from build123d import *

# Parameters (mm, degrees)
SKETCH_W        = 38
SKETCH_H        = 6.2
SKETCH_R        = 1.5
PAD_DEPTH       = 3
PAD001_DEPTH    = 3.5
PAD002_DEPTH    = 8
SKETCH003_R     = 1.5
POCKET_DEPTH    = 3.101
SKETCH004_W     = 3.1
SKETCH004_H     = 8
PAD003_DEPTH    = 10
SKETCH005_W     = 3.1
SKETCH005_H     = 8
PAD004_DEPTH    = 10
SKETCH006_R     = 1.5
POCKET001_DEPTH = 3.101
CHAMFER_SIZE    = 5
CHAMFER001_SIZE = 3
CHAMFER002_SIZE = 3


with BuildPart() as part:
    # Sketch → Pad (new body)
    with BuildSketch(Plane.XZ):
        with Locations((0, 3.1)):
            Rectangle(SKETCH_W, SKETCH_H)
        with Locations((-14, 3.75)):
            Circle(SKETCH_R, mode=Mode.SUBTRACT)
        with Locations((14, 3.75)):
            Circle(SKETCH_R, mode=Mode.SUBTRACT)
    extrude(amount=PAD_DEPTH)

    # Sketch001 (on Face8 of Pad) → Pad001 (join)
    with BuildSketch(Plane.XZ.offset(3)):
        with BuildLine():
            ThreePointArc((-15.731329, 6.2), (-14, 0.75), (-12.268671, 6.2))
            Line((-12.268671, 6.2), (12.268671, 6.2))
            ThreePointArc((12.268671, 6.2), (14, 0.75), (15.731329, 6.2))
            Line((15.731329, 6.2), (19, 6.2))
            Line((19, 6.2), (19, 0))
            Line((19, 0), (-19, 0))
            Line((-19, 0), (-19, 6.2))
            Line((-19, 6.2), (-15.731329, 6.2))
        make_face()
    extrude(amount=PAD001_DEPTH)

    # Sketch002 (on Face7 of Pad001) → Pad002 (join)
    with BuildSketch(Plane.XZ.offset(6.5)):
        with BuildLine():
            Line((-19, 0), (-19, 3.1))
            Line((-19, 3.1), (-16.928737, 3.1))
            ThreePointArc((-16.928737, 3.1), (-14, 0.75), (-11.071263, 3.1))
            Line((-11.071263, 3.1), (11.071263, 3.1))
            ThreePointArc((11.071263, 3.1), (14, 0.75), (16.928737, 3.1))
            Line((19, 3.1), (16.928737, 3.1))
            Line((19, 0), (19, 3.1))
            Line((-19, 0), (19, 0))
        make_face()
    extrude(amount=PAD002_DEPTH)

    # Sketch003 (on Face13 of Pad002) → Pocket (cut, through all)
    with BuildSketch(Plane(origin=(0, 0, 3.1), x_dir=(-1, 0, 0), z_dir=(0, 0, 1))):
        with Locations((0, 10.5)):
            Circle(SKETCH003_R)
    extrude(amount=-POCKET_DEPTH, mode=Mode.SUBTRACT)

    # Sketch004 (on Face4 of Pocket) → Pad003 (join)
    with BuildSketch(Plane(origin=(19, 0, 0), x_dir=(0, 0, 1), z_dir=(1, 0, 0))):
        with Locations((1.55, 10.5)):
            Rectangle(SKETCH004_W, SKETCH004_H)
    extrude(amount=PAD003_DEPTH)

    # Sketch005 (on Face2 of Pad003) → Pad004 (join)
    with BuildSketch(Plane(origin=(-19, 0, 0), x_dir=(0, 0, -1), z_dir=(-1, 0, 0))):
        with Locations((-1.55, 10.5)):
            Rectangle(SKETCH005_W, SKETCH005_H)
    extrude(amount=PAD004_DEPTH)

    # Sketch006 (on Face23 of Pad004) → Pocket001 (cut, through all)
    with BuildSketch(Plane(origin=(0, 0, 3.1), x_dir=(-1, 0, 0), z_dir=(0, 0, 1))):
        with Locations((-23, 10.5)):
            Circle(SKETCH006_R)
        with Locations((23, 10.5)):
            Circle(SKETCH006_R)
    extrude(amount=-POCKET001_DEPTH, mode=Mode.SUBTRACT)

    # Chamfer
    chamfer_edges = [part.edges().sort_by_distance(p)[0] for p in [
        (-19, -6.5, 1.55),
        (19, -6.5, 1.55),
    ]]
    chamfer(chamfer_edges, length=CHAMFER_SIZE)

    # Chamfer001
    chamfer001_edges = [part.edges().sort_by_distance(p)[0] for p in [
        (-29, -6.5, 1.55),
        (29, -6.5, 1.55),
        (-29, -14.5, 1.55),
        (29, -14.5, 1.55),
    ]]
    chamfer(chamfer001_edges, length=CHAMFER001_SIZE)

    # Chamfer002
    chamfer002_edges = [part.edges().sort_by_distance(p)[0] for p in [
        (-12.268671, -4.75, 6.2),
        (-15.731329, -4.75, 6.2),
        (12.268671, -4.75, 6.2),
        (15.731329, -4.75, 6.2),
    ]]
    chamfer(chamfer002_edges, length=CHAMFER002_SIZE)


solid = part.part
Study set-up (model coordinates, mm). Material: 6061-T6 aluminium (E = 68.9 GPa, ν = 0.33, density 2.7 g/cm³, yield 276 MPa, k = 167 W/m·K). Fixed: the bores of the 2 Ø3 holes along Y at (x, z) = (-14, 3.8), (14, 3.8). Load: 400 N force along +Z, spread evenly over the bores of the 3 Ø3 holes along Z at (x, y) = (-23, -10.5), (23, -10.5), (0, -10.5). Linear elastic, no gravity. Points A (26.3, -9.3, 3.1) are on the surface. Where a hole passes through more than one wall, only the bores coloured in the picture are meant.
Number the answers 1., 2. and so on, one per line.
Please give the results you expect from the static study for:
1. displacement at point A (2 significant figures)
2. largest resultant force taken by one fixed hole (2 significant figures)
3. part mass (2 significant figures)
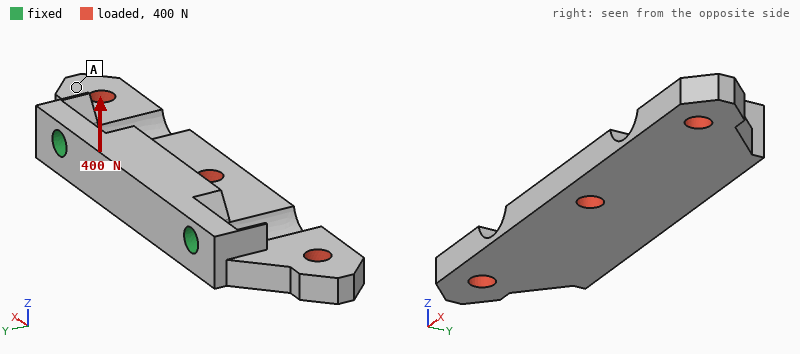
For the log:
1. 68 µm
2. 200 N
3. 6.7 g
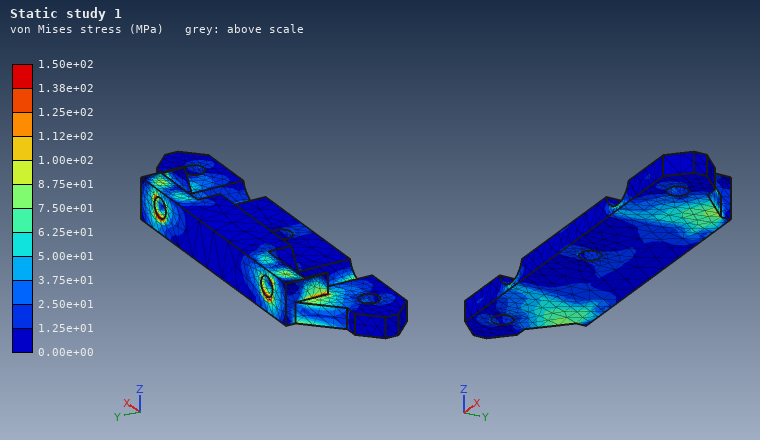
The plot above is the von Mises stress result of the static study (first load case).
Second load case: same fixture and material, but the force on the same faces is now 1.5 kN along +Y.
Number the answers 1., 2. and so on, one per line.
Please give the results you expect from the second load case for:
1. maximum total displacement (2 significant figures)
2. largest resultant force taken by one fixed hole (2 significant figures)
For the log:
1. 59 µm
2. 760 N
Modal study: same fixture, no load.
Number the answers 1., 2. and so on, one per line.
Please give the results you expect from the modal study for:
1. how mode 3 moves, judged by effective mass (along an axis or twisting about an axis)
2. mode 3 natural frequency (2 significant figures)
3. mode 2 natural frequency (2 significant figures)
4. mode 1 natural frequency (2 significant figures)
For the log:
1. along Z
2. 11 kHz
3. 9000 Hz
4. 8700 Hz
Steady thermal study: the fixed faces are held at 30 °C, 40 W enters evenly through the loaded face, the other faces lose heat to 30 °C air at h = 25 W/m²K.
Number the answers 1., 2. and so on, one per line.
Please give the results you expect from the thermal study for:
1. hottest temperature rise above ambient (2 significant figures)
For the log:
1. 46 K
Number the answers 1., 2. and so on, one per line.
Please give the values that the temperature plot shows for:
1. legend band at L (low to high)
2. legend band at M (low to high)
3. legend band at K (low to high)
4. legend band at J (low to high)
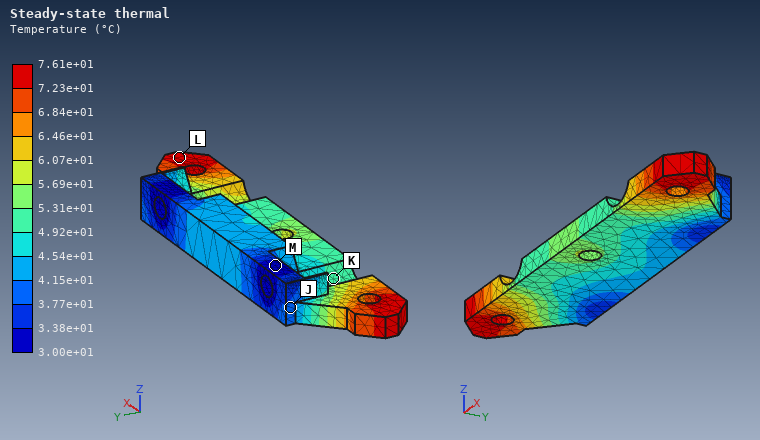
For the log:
1. 7.23e+01 to 7.61e+01 °C
2. 3.00e+01 to 3.38e+01 °C
3. 4.92e+01 to 5.31e+01 °C
4. 3.77e+01 to 4.15e+01 °C
